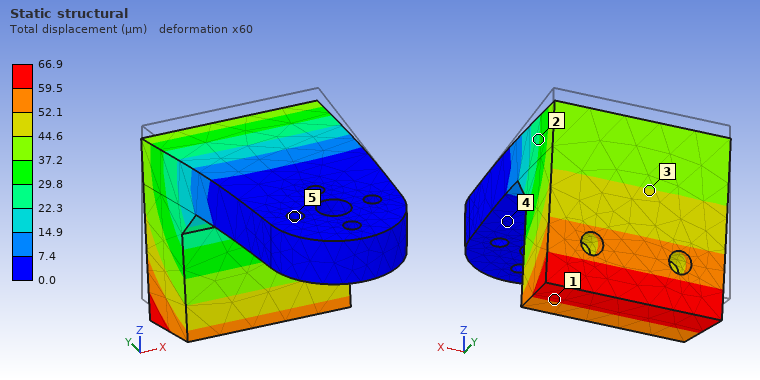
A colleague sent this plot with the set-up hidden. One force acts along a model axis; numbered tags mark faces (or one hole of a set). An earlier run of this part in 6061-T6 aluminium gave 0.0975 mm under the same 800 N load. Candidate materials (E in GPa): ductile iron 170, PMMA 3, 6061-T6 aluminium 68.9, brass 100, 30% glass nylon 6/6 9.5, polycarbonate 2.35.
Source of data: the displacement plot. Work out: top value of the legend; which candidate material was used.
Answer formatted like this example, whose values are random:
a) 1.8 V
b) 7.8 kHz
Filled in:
a) 66.9 µm
b) brass
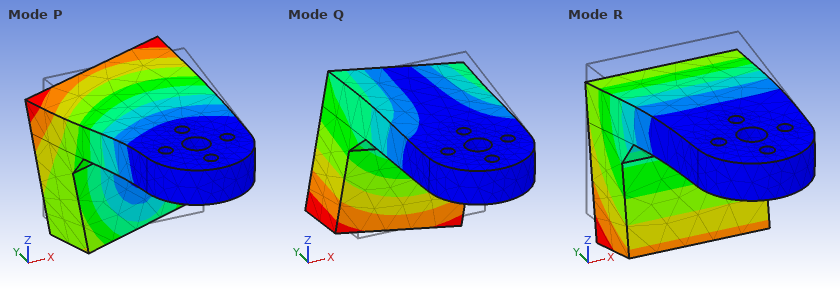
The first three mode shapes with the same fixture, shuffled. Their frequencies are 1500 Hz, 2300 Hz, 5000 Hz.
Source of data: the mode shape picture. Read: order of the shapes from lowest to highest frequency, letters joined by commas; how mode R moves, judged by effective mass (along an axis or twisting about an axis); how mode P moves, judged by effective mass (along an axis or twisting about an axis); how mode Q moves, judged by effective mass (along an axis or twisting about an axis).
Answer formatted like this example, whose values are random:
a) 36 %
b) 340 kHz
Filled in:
a) R, Q, P
b) along Z
c) along X
d) along X
